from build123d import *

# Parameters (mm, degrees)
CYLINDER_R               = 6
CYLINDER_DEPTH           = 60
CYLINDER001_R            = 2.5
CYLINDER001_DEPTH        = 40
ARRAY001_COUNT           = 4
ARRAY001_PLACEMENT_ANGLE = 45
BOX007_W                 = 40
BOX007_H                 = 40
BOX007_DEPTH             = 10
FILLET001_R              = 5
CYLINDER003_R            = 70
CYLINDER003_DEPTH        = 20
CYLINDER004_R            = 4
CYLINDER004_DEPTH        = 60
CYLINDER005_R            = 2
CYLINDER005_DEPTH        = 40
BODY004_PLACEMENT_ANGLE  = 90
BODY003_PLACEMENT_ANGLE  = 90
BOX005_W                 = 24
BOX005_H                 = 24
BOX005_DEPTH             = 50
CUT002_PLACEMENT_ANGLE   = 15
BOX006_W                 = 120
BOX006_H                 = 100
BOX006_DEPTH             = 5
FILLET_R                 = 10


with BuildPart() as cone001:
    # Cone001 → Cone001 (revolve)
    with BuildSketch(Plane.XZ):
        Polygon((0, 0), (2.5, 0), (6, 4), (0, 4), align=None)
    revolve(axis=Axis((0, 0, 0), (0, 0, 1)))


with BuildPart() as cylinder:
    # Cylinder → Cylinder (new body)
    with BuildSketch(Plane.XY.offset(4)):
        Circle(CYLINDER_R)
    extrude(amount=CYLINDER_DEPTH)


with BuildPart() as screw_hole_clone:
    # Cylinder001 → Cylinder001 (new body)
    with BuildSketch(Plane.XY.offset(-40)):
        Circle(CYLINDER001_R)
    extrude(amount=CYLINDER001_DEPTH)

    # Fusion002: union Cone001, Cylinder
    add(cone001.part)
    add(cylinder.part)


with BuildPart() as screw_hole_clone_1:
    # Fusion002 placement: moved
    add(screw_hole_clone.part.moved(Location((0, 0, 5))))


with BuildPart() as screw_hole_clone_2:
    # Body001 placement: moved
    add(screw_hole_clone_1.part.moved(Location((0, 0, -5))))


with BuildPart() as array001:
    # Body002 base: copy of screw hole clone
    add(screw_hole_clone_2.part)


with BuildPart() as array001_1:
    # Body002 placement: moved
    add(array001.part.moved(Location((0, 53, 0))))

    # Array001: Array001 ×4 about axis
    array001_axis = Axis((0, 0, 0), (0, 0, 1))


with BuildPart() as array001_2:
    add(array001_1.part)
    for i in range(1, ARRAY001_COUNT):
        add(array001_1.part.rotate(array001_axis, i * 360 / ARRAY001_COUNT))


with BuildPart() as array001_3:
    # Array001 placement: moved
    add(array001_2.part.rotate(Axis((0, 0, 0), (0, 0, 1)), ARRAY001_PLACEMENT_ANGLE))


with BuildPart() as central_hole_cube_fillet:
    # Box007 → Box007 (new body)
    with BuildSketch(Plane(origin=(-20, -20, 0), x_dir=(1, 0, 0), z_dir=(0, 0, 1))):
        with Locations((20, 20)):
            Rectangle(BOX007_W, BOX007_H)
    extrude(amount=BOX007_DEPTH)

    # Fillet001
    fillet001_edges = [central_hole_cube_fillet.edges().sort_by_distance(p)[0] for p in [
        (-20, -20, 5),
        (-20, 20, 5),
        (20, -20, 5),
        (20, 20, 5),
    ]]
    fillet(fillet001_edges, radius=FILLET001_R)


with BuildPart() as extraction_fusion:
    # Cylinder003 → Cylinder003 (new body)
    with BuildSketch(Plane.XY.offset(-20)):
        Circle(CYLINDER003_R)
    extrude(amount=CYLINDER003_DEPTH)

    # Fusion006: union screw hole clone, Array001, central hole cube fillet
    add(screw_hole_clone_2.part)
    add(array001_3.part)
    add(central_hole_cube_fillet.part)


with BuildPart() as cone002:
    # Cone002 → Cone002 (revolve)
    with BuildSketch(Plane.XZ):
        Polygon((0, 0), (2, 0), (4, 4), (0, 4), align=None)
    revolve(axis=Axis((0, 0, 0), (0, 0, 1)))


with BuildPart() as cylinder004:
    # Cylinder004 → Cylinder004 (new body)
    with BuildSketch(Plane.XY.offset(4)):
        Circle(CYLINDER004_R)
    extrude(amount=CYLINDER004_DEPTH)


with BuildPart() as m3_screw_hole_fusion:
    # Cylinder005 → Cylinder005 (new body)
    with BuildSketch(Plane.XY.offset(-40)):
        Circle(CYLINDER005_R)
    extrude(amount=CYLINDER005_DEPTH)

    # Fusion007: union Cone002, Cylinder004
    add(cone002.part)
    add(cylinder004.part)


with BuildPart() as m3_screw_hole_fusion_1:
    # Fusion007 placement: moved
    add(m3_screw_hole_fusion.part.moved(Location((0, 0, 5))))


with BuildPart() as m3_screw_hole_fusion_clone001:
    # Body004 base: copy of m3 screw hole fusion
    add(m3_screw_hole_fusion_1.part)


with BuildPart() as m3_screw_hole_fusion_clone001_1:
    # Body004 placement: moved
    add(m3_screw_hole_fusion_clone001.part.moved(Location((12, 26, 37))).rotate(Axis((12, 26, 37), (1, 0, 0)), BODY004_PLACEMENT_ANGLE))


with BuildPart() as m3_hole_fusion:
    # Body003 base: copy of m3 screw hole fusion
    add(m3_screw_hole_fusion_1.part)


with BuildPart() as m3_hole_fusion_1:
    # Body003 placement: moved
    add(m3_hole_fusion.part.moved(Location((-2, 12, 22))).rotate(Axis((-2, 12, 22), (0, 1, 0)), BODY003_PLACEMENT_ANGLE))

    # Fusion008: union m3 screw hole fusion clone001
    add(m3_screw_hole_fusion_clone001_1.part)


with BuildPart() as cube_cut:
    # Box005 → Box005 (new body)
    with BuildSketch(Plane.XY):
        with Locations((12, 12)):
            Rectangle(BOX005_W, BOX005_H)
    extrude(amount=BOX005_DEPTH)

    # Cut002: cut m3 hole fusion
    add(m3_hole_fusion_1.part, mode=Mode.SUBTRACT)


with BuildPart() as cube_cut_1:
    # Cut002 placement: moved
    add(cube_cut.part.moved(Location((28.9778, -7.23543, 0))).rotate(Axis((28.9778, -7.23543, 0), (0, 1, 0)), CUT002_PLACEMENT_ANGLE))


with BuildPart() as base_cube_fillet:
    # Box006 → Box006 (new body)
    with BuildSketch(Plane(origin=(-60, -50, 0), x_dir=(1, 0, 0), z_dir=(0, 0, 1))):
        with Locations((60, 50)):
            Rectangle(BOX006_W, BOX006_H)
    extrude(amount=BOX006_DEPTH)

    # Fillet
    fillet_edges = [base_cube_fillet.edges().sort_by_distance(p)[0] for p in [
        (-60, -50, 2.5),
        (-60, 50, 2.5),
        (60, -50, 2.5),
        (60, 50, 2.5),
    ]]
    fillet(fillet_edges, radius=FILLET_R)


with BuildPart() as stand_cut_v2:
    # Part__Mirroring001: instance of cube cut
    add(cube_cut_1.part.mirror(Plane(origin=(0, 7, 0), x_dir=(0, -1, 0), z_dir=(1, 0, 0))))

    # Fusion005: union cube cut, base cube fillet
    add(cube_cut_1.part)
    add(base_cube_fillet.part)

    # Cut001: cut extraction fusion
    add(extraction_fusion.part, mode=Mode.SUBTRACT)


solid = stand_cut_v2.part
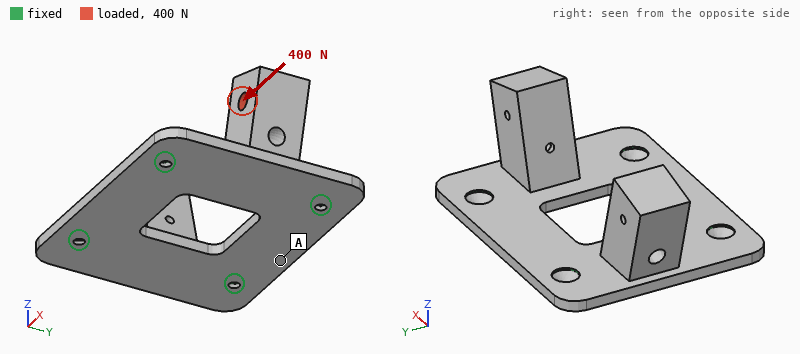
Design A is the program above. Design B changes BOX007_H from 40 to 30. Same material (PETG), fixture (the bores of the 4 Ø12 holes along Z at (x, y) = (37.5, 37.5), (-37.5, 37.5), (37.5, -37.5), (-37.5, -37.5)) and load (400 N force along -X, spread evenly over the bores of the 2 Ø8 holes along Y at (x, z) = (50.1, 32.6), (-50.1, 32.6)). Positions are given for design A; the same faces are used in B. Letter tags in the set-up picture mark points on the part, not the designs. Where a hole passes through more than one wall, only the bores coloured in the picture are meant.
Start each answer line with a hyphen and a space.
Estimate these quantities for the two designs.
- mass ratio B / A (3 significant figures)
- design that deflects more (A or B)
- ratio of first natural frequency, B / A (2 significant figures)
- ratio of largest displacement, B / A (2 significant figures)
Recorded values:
- 1.02
- A
- 1.0
- 0.91
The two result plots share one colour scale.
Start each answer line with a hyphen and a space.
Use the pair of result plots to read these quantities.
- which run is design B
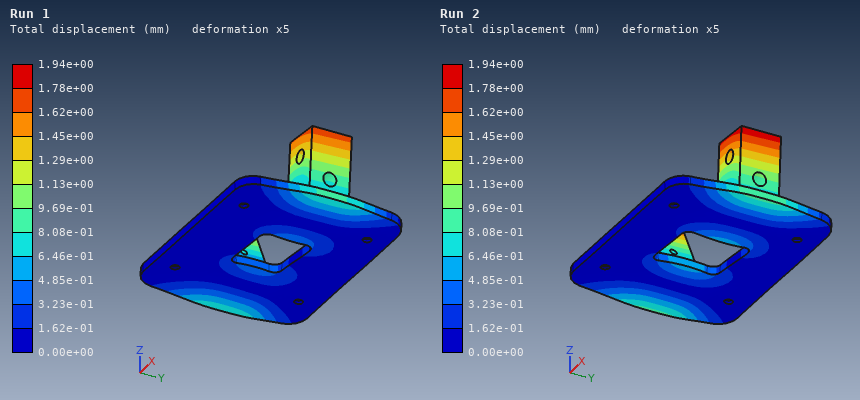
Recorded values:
- Run 1
